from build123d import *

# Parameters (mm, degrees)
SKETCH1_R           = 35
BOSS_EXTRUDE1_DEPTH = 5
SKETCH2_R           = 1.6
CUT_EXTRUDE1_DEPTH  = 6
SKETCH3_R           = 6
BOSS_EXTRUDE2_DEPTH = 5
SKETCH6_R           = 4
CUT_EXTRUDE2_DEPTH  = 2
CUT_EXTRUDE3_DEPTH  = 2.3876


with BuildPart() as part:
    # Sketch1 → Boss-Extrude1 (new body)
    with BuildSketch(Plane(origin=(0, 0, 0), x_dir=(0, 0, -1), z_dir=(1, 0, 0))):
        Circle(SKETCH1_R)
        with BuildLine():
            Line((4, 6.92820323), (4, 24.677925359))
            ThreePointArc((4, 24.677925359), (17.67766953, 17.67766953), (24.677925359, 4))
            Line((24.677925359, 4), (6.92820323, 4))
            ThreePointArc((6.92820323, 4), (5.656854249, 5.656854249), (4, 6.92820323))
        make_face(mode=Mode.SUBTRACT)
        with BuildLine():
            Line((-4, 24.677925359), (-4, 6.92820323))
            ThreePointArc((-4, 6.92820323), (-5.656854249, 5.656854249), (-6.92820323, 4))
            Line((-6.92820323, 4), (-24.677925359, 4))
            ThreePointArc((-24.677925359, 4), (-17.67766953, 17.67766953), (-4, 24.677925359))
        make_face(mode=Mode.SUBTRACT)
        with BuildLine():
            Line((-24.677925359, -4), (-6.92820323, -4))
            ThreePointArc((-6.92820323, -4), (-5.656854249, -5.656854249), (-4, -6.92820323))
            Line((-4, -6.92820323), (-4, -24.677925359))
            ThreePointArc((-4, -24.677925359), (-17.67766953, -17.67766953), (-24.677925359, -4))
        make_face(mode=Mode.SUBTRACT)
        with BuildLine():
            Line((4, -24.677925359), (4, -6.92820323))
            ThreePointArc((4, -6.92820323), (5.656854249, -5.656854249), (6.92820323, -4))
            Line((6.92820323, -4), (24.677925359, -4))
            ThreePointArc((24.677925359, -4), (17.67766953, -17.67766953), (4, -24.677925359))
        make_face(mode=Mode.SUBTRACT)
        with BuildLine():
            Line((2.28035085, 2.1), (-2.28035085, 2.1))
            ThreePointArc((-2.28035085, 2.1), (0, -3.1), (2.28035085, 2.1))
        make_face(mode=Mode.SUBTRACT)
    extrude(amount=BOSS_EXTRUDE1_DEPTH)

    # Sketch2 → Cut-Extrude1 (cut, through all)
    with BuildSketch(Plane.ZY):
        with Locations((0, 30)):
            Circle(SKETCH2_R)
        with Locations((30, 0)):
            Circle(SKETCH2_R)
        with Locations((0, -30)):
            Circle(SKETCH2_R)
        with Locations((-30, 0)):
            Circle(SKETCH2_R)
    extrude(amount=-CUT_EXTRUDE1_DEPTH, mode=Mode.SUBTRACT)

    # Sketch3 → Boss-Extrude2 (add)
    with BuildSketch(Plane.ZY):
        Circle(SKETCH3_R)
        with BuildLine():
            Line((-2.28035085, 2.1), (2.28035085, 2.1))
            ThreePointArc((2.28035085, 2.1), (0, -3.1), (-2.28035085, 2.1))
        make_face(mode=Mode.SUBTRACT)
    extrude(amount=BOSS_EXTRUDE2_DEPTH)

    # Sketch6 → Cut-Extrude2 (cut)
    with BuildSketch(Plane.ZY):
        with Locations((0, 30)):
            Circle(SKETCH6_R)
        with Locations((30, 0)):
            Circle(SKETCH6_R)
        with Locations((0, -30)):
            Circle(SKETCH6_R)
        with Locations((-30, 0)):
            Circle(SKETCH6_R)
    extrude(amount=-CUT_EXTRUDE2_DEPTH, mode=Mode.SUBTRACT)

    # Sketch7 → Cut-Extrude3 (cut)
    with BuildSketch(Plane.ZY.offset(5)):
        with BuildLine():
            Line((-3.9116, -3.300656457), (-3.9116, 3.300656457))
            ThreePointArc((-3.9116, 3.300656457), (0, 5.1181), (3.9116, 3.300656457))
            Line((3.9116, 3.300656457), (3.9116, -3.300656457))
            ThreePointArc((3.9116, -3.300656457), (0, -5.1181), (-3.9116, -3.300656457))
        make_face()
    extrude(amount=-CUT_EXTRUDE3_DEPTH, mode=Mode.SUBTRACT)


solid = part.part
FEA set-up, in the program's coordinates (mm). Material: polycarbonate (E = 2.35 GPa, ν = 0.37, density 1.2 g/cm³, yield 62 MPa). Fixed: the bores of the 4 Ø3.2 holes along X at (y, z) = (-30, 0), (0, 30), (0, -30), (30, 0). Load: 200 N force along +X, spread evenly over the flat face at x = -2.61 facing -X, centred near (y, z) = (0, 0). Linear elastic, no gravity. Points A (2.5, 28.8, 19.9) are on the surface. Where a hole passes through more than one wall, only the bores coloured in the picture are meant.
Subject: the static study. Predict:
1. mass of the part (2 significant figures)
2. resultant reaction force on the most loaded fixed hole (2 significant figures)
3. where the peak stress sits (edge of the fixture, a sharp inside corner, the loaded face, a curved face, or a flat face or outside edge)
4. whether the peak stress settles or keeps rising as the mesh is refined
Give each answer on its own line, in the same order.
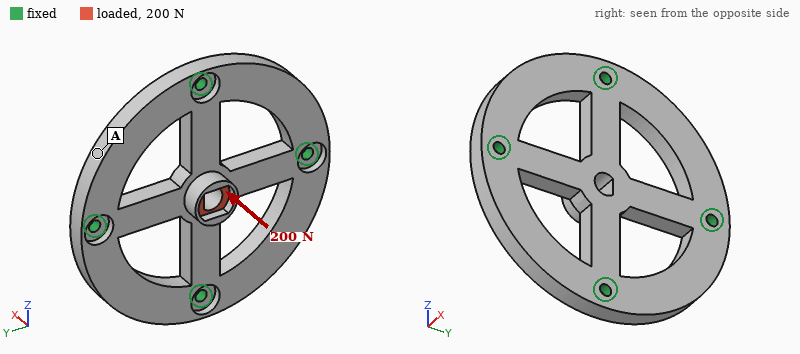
15 g
88 N
edge of the fixture
keeps rising
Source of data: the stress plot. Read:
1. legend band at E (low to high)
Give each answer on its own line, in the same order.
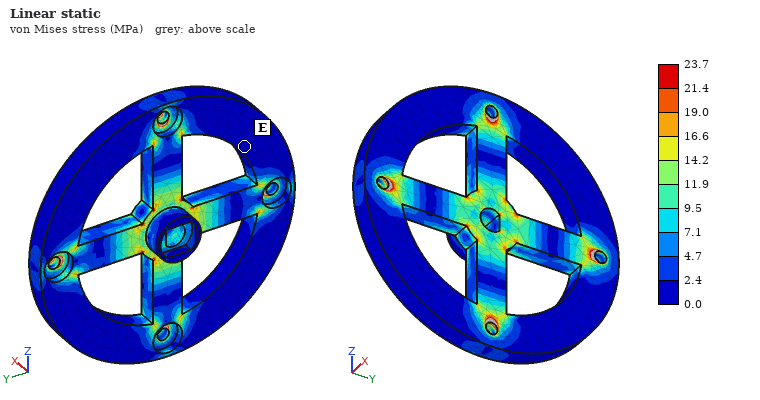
0.0 to 2.4 MPa
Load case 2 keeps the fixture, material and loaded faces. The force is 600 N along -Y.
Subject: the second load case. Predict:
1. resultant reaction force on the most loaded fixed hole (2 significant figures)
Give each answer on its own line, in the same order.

280 N
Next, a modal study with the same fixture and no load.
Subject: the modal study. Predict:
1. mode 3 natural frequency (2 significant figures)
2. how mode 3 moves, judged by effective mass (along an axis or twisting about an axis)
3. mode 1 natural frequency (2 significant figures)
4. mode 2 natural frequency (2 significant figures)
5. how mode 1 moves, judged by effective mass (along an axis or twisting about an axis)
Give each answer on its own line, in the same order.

2300 Hz
twisting about Y
2000 Hz
2100 Hz
along X
